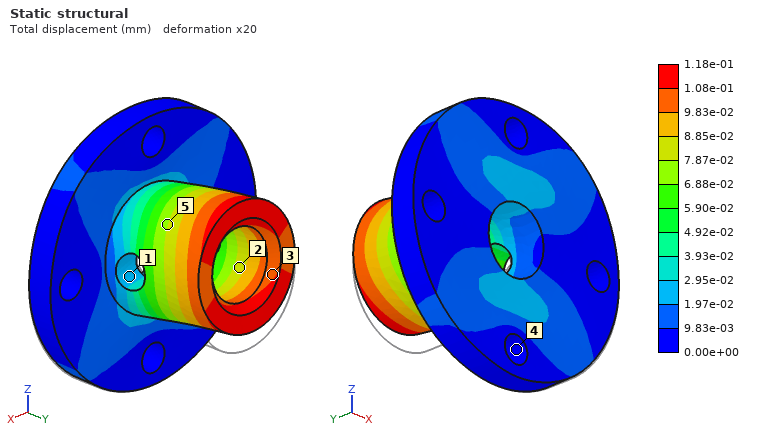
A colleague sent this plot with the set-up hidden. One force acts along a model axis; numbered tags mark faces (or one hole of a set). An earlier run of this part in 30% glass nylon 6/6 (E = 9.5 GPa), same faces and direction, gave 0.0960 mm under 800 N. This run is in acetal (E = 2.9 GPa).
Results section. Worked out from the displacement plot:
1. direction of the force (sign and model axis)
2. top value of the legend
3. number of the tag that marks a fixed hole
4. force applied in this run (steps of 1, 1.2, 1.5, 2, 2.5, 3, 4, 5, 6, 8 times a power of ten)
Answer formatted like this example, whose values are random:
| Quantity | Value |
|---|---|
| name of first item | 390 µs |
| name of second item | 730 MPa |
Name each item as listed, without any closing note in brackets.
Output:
| Quantity | Value |
|---|---|
| direction of the force | +Z |
| top value of the legend | 1.18e-01 mm |
| number of the tag that marks a fixed hole | 4 |
| force applied in this run | 300 N |
